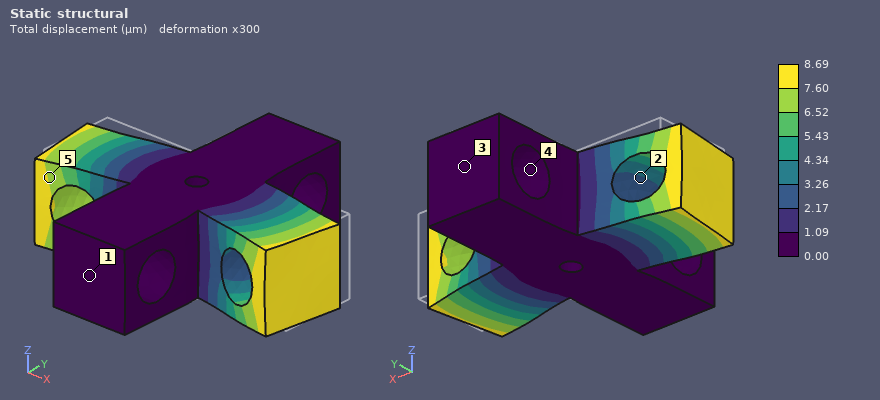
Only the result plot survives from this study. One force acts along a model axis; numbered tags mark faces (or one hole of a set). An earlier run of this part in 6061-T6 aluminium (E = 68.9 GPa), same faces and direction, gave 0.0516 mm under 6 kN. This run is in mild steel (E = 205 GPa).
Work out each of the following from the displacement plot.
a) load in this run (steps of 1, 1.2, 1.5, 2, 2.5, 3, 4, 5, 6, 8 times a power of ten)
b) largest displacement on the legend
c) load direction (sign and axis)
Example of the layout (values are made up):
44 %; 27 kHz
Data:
3 kN; 8.69 µm; -Y
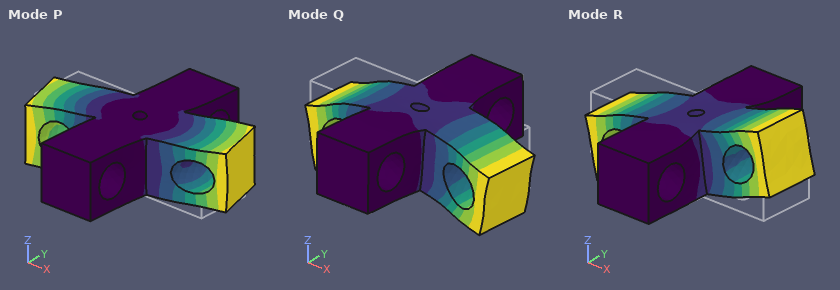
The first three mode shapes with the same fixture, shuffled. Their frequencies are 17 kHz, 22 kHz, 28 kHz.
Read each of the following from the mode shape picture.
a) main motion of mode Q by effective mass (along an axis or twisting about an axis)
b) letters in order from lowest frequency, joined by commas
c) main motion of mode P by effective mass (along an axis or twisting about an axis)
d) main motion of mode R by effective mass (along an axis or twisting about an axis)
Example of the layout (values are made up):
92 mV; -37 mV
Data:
along Z; R, Q, P; twisting about Z; twisting about Y
